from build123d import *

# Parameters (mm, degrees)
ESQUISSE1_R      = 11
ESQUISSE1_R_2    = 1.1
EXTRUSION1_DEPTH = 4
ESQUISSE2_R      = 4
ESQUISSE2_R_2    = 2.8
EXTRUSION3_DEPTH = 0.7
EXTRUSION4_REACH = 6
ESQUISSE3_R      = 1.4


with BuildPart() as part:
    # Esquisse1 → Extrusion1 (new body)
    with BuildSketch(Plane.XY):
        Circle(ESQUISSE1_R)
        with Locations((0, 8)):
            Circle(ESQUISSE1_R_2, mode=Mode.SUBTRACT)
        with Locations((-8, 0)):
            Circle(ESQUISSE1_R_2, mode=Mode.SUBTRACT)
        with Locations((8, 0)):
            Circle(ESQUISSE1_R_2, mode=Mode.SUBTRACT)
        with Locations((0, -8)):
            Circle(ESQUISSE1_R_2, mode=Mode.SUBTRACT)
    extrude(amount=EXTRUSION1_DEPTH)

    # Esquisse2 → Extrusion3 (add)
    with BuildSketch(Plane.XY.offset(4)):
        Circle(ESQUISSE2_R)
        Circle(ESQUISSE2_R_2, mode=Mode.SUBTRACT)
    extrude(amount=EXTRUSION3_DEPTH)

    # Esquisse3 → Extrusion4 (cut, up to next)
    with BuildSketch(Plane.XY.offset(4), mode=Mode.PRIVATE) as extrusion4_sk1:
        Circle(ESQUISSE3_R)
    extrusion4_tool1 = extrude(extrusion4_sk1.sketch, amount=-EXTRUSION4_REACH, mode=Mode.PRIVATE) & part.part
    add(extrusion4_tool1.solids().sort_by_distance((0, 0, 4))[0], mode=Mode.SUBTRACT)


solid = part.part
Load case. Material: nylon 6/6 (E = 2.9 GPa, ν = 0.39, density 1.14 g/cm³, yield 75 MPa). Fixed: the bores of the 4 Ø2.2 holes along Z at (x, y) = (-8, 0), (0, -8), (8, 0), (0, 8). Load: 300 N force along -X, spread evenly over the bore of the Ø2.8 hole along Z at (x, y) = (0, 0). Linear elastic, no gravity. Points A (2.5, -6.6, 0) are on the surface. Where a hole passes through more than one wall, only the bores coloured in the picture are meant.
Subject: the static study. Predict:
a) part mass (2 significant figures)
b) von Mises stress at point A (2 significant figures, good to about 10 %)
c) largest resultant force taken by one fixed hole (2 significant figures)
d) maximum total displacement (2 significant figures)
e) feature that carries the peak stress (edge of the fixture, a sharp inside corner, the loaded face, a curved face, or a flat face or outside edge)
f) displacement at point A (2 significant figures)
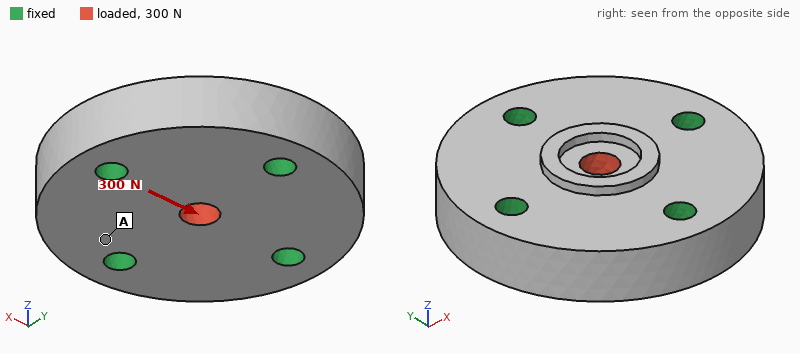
1.7 g
1.6 MPa
100 N
14 µm
the loaded face
2.6 µm
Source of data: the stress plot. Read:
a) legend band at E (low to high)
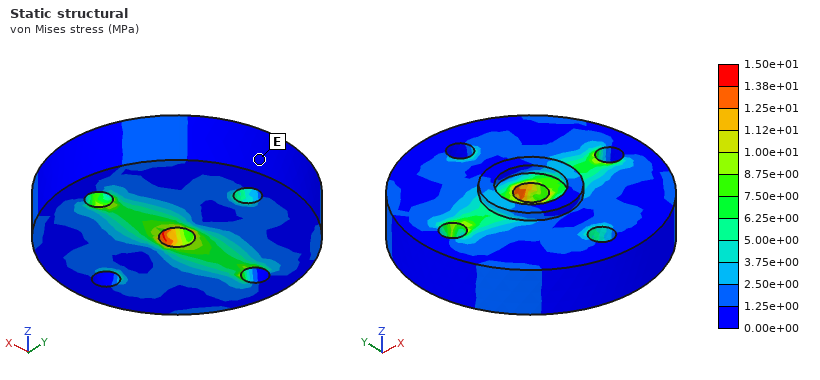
0.00e+00 to 1.25e+00 MPa
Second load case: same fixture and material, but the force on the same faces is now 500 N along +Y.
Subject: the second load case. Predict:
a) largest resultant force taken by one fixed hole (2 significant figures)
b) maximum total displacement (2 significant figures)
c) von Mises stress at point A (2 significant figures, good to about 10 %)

170 N
24 µm
3.5 MPa
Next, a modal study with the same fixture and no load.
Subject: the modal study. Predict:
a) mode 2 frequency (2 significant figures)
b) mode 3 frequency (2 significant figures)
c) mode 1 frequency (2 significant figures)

26 kHz
26 kHz
25 kHz
